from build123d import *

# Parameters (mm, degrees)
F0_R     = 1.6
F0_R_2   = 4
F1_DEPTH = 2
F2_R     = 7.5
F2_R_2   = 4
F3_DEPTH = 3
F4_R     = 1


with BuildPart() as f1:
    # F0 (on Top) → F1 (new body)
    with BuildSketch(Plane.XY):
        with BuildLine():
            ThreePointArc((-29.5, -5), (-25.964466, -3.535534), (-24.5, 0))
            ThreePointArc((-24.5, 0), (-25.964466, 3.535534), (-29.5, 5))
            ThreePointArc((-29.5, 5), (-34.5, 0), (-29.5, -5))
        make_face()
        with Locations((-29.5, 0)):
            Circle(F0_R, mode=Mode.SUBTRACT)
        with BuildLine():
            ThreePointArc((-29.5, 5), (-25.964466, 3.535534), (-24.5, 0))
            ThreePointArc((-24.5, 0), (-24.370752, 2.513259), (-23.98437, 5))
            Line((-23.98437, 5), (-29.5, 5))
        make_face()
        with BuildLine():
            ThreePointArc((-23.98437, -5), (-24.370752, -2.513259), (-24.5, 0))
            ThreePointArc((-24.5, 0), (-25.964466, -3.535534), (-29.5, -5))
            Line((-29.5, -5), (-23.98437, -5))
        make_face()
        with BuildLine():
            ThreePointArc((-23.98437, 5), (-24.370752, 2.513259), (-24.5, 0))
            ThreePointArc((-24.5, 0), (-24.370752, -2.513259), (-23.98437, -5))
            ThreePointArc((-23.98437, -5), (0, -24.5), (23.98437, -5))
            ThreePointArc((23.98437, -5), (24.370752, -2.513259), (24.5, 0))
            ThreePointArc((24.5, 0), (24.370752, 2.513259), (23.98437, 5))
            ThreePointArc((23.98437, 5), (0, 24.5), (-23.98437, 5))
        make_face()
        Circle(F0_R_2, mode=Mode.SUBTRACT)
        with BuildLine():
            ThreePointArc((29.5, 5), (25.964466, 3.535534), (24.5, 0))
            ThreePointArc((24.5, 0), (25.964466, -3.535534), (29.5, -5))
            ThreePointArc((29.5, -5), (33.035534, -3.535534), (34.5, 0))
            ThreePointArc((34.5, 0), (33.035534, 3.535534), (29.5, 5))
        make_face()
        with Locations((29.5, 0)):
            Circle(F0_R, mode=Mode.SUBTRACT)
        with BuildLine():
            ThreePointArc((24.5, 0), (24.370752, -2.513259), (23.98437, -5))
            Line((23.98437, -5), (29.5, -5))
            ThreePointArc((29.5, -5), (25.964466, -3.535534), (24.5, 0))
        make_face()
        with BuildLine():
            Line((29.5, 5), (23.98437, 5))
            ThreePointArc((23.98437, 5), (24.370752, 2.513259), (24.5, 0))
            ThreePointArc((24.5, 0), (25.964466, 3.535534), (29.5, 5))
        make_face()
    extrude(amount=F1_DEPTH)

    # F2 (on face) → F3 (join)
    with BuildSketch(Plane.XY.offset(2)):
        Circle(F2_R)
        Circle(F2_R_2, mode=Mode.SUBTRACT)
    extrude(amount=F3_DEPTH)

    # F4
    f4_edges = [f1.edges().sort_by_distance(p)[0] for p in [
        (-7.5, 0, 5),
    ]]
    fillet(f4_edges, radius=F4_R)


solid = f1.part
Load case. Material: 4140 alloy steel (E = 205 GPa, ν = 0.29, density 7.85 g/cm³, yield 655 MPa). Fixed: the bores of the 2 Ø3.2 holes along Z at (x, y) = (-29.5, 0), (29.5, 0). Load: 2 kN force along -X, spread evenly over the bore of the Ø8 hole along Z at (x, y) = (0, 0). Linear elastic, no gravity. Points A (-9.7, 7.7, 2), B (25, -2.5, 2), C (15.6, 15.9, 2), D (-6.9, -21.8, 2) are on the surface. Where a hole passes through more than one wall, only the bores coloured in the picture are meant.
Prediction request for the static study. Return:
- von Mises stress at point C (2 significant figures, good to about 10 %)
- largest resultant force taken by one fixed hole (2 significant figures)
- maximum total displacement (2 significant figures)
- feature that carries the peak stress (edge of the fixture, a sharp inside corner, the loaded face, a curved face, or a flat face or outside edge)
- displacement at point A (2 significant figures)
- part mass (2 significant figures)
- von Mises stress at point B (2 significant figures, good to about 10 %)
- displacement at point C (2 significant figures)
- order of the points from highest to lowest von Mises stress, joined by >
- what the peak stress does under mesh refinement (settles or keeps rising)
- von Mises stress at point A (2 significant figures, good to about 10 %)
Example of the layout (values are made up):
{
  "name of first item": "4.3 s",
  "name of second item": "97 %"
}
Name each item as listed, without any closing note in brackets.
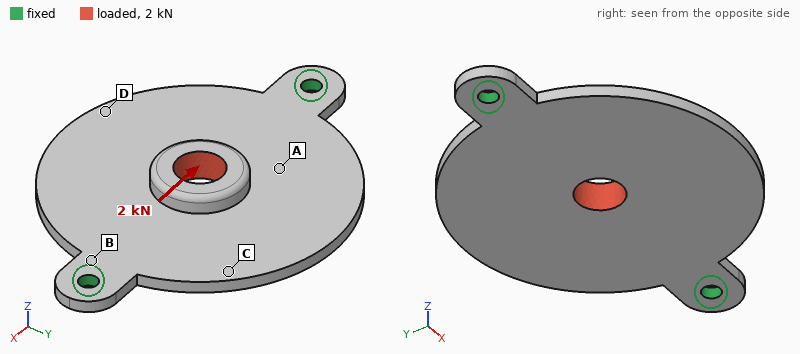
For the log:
{
  "von Mises stress at point C": "17 MPa",
  "largest resultant force taken by one fixed hole": "1.0 kN",
  "maximum total displacement": "14 µm",
  "feature that carries the peak stress": "edge of the fixture",
  "displacement at point A": "11 µm",
  "part mass": "34 g",
  "von Mises stress at point B": "31 MPa",
  "displacement at point C": "11 µm",
  "order of the points from highest to lowest von Mises stress, joined by >": "A > B > C > D",
  "what the peak stress does under mesh refinement": "keeps rising",
  "von Mises stress at point A": "46 MPa"
}
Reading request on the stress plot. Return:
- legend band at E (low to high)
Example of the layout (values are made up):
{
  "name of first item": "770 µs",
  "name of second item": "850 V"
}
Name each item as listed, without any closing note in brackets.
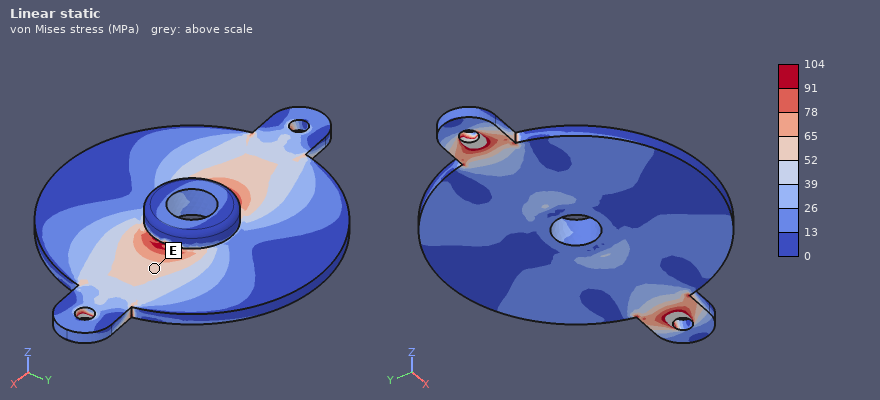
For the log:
{
  "legend band at E": "52 to 65 MPa"
}
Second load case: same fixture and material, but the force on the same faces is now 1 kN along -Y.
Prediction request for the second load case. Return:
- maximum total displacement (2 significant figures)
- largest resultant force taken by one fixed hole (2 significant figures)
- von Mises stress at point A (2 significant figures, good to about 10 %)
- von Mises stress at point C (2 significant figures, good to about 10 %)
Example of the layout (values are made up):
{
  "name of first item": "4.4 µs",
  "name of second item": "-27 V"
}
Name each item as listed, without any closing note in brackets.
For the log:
{
  "maximum total displacement": "0.10 mm",
  "largest resultant force taken by one fixed hole": "500 N",
  "von Mises stress at point A": "24 MPa",
  "von Mises stress at point C": "15 MPa"
}
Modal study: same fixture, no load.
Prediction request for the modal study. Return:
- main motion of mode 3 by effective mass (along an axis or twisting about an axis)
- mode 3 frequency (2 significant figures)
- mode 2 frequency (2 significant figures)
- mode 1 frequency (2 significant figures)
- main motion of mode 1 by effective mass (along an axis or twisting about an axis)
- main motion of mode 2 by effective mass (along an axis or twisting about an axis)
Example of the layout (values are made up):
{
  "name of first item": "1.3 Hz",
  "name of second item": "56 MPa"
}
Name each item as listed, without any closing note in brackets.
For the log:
{
  "main motion of mode 3 by effective mass": "twisting about Y",
  "mode 3 frequency": "5700 Hz",
  "mode 2 frequency": "2100 Hz",
  "mode 1 frequency": "1500 Hz",
  "main motion of mode 1 by effective mass": "twisting about X",
  "main motion of mode 2 by effective mass": "along Z"
}
